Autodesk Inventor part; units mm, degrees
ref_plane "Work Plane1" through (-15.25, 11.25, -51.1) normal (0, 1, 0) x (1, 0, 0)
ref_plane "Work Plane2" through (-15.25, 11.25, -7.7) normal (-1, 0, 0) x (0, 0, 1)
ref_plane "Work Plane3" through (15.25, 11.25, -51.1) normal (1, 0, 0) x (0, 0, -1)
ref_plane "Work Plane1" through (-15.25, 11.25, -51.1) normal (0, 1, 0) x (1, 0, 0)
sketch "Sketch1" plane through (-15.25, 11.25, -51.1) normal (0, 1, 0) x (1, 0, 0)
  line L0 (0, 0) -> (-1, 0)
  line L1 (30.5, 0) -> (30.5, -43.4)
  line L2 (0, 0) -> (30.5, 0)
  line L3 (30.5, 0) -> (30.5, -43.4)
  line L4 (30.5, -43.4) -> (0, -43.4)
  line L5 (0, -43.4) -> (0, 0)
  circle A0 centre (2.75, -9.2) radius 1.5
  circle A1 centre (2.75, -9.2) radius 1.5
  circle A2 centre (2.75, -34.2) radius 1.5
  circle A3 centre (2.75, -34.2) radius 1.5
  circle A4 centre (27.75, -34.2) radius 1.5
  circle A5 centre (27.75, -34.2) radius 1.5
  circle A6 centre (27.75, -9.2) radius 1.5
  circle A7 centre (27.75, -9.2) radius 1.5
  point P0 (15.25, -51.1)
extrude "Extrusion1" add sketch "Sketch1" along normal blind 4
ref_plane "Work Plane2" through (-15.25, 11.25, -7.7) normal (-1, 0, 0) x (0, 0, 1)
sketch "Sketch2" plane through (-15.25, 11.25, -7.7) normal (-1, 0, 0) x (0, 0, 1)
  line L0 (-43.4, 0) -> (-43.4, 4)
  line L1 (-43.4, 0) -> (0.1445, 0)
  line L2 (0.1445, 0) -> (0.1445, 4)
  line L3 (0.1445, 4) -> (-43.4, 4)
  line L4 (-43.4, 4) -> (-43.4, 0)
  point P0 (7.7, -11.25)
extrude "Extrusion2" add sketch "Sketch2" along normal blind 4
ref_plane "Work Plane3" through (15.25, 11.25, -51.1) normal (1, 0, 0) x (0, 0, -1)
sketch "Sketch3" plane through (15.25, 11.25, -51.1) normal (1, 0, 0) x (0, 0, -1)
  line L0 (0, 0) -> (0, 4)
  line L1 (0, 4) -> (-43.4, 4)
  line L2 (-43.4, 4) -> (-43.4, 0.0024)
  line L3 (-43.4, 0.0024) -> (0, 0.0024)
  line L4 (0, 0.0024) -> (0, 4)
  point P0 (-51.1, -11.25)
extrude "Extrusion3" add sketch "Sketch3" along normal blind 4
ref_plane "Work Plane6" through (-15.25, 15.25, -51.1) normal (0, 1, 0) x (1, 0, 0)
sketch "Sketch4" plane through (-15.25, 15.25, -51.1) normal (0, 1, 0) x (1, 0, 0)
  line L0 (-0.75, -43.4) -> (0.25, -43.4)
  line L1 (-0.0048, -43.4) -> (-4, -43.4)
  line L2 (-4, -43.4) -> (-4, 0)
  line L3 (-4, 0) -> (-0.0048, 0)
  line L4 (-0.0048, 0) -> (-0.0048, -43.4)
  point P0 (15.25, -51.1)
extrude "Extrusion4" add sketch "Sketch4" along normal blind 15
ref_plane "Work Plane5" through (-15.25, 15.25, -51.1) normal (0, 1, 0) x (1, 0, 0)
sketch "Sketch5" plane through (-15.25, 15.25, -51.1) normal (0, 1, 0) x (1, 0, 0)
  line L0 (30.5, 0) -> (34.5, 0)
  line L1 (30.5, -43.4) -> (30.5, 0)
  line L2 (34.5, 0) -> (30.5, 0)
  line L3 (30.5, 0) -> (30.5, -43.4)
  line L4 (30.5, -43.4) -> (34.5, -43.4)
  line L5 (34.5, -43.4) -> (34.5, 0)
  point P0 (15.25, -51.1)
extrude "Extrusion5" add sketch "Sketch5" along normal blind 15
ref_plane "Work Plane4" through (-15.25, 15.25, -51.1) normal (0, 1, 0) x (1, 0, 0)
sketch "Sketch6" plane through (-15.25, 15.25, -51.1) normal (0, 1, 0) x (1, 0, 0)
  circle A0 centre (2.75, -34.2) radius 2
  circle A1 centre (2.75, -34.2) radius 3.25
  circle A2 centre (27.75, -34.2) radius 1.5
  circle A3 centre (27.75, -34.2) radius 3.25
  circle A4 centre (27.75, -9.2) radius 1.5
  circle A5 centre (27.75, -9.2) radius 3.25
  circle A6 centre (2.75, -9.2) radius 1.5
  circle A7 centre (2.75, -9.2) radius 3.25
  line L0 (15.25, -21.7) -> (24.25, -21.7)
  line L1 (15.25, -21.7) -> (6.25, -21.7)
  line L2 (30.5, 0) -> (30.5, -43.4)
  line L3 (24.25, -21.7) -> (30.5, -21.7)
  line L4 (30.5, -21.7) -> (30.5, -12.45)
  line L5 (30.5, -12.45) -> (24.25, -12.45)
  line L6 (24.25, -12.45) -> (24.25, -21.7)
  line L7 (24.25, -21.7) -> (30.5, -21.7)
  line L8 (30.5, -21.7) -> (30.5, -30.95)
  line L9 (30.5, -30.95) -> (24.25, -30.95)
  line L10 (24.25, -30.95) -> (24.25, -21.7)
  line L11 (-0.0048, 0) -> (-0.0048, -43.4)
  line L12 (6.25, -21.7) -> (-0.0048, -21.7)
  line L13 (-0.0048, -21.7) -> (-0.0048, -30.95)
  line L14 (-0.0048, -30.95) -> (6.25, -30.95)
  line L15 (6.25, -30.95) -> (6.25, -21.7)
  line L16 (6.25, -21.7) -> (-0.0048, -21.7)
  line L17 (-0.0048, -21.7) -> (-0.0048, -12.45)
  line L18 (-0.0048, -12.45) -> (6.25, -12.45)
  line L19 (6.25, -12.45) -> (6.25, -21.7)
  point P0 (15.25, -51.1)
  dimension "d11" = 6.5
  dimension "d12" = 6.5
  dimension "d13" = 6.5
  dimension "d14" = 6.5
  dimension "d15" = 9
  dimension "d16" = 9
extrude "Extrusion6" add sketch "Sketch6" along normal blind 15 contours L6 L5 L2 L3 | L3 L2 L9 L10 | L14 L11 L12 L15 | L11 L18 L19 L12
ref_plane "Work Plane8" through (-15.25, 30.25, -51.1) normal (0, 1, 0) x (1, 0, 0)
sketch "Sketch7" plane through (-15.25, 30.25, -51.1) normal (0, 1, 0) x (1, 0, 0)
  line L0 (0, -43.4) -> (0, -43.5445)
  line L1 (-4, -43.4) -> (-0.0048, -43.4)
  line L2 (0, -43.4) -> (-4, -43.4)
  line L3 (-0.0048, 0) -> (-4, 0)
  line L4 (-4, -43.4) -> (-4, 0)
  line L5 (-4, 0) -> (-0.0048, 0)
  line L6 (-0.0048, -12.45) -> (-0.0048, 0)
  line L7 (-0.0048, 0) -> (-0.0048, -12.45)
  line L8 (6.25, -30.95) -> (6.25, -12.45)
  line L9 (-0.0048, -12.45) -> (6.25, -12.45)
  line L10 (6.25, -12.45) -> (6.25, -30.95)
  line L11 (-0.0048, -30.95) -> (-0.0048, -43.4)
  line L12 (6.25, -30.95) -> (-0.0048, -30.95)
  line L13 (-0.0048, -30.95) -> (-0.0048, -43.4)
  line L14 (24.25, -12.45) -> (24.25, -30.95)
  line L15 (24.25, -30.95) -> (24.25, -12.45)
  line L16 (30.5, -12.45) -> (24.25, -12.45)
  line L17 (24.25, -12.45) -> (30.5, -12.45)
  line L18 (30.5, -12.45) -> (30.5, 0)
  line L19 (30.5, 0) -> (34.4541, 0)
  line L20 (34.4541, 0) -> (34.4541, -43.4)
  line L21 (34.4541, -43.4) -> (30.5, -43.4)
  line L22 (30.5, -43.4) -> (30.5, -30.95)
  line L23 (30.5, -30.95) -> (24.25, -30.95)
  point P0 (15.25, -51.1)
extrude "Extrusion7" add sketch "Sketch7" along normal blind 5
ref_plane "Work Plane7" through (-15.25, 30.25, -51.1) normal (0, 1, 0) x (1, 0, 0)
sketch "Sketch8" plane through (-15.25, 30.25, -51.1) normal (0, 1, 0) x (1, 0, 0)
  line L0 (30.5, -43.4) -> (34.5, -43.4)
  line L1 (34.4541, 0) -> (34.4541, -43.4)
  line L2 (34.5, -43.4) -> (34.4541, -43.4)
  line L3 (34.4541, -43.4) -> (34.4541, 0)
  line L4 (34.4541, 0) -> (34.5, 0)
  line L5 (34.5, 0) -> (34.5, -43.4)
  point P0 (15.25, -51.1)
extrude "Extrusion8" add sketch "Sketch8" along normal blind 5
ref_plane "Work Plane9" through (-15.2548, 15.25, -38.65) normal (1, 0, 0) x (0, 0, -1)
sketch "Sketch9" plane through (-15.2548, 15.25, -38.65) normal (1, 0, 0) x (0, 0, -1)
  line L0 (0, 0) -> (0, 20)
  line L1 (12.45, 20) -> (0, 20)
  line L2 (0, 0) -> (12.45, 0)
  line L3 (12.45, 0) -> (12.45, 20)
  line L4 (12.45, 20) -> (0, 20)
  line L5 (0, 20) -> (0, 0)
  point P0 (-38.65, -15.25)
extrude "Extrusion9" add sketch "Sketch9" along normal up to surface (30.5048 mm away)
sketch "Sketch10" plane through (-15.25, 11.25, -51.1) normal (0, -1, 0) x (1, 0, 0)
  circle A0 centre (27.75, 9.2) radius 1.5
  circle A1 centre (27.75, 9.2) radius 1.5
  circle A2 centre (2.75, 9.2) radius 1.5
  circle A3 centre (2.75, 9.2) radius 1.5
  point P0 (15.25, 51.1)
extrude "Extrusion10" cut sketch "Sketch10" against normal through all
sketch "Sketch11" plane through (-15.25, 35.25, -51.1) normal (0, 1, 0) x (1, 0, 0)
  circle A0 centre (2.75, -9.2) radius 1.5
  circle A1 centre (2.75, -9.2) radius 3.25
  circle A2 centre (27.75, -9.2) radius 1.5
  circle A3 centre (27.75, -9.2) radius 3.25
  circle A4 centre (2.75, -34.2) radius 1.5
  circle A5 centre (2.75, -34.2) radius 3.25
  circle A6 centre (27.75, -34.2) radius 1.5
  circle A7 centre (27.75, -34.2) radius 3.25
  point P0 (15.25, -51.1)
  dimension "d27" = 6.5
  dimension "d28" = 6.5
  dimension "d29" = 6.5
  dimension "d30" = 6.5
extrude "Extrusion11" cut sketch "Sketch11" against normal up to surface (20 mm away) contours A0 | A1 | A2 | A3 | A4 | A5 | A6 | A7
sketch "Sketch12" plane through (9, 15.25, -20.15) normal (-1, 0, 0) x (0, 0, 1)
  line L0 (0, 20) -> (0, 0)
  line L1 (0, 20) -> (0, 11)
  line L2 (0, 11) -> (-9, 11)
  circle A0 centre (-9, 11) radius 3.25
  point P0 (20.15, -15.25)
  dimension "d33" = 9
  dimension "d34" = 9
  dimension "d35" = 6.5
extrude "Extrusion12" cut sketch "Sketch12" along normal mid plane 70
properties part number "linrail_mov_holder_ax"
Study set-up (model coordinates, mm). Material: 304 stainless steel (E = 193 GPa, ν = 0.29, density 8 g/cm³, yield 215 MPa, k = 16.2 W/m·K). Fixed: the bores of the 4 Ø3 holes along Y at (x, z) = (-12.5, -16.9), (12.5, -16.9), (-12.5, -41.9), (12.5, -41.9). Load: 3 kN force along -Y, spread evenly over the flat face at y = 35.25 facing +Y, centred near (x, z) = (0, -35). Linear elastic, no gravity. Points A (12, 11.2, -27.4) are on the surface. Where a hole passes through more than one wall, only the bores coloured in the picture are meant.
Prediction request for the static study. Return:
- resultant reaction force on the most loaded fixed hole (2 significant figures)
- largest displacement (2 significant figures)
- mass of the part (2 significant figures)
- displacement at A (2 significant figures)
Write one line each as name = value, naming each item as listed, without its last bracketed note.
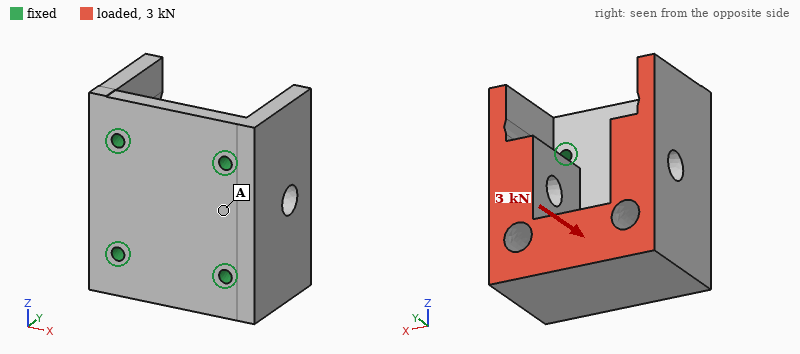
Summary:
resultant reaction force on the most loaded fixed hole = 1.1 kN
largest displacement = 1.6 µm
mass of the part = 190 g
displacement at A = 0.88 µm
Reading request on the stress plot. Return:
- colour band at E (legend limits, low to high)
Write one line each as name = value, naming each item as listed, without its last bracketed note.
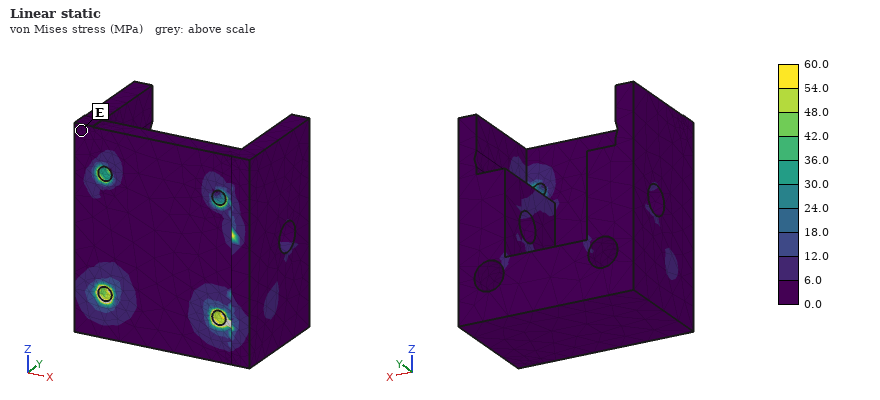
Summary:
colour band at E = 0.0 to 6.0 MPa
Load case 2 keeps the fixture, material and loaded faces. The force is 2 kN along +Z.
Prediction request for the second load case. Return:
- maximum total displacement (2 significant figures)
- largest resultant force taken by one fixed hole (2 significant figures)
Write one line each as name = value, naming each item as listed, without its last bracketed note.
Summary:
maximum total displacement = 5.8 µm
largest resultant force taken by one fixed hole = 1.0 kN
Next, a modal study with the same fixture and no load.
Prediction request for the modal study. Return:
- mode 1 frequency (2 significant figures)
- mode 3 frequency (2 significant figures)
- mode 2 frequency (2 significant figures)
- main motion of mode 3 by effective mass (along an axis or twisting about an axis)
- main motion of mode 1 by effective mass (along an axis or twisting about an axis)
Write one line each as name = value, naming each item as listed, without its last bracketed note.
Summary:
mode 1 frequency = 10 kHz
mode 3 frequency = 13 kHz
mode 2 frequency = 11 kHz
main motion of mode 3 by effective mass = along Z
main motion of mode 1 by effective mass = along X
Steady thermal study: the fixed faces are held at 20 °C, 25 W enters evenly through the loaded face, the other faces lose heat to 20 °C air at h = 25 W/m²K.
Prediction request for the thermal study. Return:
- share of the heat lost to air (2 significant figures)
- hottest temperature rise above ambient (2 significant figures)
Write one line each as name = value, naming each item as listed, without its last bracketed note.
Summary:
share of the heat lost to air = 24 %
hottest temperature rise above ambient = 55 K
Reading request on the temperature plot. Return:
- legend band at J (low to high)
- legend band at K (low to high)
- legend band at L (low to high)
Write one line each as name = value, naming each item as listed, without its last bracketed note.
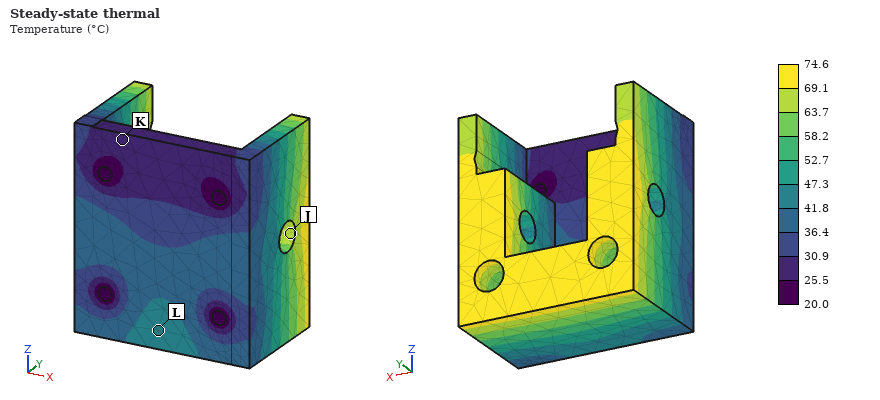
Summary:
legend band at J = 63.7 to 69.1 °C
legend band at K = 25.5 to 30.9 °C
legend band at L = 41.8 to 47.3 °C
